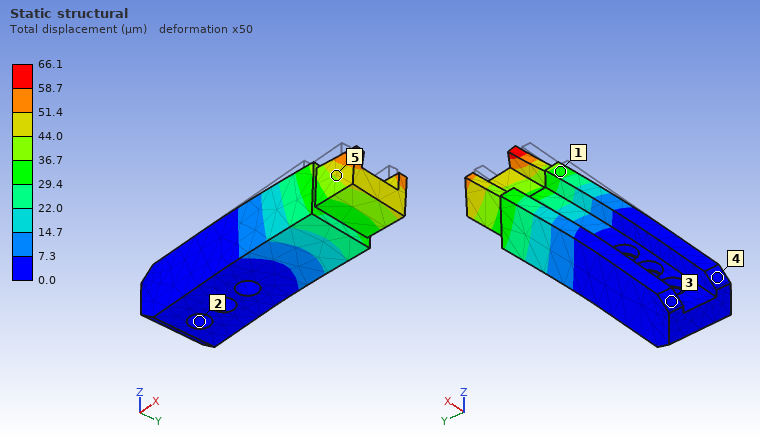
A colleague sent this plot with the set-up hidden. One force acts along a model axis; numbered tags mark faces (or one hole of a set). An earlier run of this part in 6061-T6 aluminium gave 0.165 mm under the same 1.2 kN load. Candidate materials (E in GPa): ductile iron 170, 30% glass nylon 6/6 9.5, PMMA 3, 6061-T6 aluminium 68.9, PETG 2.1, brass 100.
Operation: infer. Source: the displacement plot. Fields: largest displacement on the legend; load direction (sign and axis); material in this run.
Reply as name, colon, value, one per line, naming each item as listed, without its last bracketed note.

largest displacement on the legend: 66.1 µm
load direction: +Y
material in this run: ductile iron
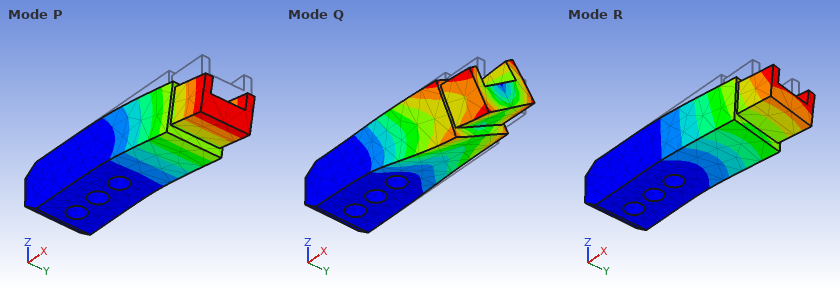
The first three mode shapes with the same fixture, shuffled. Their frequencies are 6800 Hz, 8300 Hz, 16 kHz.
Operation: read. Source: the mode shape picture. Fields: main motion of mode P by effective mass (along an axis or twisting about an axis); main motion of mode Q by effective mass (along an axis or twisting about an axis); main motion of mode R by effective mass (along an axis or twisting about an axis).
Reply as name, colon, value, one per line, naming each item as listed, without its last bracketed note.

main motion of mode P by effective mass: along Z
main motion of mode Q by effective mass: twisting about X
main motion of mode R by effective mass: along Y
